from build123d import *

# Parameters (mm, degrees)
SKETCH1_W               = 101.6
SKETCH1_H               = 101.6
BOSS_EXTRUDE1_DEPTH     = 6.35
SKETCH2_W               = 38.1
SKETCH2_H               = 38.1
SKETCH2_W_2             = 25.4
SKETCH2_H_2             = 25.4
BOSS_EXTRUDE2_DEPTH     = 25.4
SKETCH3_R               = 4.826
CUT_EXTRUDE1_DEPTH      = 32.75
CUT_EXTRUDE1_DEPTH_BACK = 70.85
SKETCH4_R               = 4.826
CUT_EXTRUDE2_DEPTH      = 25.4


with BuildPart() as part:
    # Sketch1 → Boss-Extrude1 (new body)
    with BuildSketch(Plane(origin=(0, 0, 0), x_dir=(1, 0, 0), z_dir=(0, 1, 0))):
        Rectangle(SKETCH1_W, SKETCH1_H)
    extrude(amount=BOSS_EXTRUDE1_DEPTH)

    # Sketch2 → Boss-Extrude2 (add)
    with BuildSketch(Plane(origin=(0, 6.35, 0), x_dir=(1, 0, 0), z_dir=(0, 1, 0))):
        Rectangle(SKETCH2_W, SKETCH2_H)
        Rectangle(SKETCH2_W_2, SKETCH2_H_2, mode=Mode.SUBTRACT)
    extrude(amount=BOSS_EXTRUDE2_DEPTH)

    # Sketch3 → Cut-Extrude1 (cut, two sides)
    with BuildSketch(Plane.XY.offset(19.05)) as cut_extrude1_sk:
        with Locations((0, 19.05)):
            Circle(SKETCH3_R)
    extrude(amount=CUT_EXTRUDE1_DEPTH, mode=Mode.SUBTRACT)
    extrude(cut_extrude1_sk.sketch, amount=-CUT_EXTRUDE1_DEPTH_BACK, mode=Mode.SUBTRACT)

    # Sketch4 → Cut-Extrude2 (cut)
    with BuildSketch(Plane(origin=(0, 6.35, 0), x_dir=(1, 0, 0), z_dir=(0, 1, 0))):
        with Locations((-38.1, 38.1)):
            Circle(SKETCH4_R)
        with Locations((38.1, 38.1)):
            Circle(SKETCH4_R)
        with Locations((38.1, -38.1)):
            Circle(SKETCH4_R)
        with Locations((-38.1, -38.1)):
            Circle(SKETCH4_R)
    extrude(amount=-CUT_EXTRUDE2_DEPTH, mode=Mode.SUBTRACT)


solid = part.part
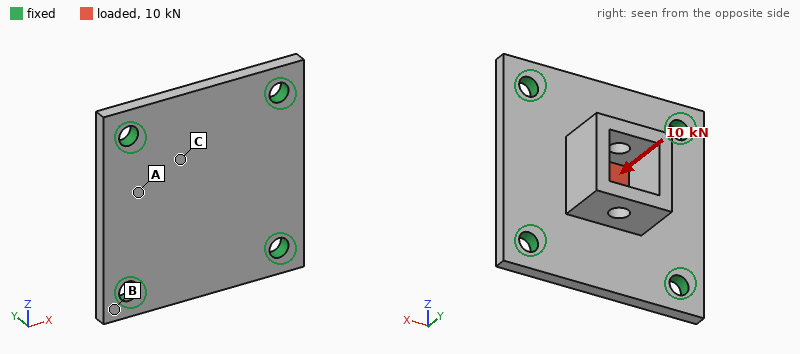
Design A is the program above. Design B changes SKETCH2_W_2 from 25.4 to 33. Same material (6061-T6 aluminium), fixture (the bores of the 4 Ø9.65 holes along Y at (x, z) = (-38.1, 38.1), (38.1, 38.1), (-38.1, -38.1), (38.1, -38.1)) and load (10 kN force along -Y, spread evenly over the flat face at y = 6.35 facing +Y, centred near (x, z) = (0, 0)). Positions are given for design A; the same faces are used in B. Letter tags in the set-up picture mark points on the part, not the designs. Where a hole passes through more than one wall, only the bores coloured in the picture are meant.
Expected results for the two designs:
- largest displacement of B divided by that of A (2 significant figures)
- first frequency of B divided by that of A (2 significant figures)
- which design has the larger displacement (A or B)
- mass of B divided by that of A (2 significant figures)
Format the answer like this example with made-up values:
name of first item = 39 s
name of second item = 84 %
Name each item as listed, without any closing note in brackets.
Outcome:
largest displacement of B divided by that of A = 1.1
first frequency of B divided by that of A = 1.0
which design has the larger displacement = B
mass of B divided by that of A = 0.94
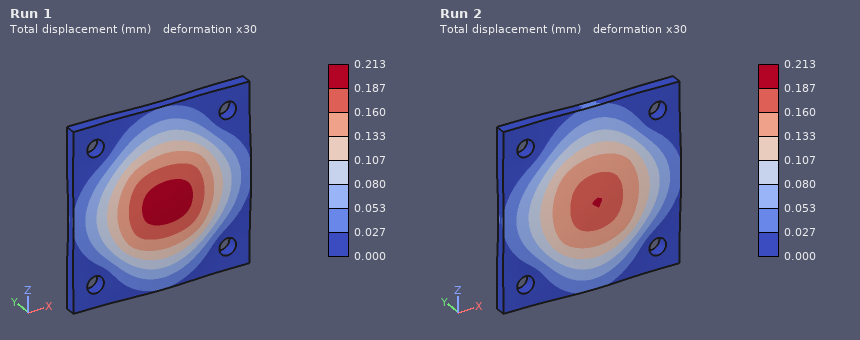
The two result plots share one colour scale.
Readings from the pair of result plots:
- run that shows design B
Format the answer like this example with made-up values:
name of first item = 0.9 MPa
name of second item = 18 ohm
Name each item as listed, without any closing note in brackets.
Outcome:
run that shows design B = Run 1
